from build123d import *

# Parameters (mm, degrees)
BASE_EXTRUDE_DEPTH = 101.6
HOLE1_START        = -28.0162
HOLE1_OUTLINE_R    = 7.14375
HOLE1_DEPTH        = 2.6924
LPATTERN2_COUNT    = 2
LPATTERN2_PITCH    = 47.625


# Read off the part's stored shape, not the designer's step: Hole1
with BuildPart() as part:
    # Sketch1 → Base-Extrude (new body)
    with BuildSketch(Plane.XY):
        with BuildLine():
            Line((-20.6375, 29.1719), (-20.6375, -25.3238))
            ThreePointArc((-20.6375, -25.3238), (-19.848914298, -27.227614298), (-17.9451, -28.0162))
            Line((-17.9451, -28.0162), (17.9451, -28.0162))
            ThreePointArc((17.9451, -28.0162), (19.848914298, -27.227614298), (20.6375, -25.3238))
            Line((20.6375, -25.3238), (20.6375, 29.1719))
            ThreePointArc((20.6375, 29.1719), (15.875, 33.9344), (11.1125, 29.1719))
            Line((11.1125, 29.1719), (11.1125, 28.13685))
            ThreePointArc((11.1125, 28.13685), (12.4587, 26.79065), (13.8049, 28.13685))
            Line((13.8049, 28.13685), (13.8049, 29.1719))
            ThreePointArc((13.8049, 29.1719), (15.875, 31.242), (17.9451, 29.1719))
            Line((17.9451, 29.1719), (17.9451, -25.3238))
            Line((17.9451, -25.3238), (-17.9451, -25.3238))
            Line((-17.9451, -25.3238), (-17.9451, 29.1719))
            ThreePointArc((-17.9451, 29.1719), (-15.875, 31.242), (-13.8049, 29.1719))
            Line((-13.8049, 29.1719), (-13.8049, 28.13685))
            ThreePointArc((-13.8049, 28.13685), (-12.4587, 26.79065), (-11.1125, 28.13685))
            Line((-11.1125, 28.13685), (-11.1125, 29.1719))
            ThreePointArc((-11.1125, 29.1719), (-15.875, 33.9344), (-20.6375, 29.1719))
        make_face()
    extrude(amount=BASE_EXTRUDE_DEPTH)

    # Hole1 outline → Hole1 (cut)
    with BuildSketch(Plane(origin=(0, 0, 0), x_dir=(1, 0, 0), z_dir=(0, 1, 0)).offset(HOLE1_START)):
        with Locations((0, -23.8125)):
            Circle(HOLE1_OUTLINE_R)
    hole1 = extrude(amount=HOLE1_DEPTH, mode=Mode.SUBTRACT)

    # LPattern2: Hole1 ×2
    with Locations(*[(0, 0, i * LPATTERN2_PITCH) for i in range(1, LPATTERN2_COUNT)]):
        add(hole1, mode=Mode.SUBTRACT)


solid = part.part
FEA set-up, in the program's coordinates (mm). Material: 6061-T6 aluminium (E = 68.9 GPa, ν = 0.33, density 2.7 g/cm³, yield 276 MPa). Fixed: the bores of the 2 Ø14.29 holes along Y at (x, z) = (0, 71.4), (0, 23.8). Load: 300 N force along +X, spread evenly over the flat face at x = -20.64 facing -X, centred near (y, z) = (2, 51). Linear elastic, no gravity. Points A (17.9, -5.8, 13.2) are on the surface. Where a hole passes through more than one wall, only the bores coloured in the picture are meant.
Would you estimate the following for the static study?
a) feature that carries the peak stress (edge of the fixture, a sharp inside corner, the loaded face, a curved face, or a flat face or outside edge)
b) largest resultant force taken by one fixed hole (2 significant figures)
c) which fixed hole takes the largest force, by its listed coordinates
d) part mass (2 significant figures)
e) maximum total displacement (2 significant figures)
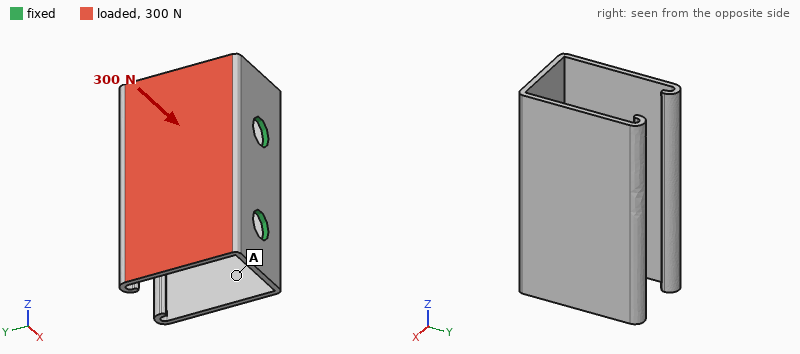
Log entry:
a flat face or outside edge
160 N
(0, 71.4)
130 g
1.2 mm
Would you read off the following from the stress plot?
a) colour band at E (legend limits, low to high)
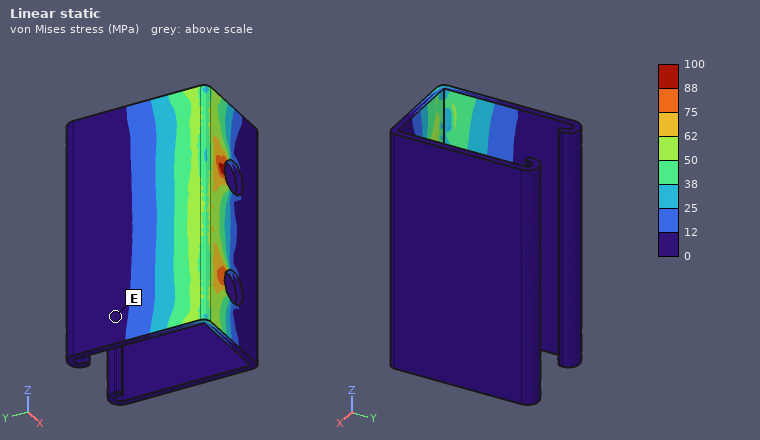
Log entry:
0 to 12 MPa
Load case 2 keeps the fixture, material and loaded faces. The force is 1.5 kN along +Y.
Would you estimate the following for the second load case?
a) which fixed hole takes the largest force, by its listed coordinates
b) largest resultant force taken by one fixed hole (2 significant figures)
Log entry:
(0, 71.4)
830 N
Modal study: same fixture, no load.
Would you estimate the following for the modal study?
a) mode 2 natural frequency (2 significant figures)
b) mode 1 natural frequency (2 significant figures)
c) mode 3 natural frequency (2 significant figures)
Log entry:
380 Hz
380 Hz
750 Hz
